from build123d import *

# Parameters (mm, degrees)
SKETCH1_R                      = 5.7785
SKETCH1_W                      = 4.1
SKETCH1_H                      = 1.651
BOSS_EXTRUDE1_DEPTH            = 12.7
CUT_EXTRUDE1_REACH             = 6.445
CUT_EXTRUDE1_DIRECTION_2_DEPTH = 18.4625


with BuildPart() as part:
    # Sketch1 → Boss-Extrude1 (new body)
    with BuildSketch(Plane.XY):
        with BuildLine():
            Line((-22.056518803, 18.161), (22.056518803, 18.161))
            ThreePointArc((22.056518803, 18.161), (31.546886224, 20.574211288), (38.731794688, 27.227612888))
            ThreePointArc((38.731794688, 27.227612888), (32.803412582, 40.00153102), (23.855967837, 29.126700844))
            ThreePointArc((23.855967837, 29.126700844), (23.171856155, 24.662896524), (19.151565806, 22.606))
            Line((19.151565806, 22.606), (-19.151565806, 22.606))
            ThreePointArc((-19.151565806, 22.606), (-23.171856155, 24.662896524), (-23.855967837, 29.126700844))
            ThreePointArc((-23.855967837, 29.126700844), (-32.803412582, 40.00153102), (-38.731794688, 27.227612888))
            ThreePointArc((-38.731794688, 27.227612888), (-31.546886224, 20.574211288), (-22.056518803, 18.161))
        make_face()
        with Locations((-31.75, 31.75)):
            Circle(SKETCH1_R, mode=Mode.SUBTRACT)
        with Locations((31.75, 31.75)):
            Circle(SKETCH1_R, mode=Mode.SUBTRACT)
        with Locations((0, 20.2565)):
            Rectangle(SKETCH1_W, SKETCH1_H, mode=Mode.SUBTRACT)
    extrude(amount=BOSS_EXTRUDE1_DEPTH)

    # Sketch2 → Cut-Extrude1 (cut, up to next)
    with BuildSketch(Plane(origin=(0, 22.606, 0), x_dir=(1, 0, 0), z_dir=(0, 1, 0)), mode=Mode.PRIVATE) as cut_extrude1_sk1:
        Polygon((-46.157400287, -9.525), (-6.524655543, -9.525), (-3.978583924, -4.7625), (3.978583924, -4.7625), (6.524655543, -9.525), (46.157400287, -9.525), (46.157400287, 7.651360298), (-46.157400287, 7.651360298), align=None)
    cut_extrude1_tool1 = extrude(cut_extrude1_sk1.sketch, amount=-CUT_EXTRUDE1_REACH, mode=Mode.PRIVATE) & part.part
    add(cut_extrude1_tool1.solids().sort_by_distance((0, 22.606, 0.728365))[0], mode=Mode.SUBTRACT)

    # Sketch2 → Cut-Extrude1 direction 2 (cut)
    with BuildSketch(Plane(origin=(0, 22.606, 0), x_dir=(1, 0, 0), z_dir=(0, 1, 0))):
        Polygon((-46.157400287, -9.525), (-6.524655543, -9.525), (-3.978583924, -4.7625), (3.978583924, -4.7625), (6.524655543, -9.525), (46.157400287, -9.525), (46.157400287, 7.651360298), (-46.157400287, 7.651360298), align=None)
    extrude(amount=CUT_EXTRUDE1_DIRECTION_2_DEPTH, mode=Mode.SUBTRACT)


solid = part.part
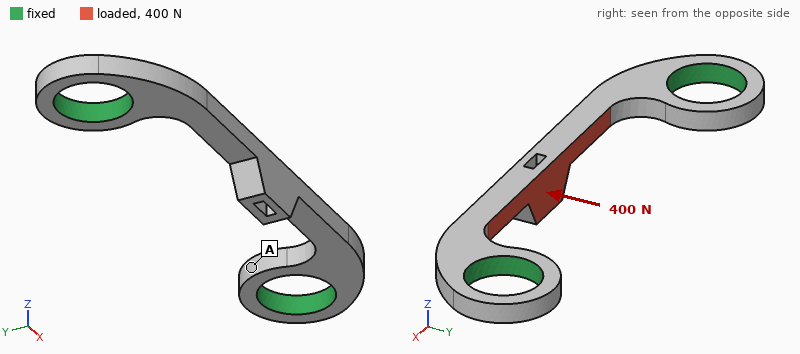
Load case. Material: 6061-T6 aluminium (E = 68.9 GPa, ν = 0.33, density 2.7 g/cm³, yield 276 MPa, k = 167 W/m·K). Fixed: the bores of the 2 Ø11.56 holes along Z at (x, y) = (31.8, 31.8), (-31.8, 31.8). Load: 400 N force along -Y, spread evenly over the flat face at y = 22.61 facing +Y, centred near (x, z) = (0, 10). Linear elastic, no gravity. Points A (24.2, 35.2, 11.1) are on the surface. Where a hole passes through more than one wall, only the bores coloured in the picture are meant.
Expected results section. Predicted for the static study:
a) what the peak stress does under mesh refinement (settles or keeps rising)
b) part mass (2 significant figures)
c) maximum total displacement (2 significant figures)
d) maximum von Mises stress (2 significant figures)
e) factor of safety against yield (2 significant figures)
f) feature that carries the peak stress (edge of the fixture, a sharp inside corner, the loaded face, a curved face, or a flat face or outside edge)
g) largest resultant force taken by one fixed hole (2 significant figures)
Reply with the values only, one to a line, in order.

settles
5.2 g
0.15 mm
170 MPa
1.7
a curved face
270 N
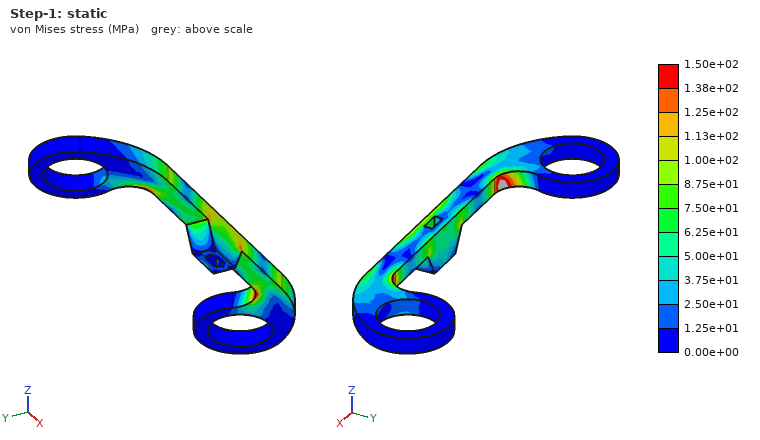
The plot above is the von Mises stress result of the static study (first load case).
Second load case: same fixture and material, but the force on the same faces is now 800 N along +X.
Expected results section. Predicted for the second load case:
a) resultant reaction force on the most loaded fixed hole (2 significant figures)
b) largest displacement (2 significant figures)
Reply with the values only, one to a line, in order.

400 N
30 µm
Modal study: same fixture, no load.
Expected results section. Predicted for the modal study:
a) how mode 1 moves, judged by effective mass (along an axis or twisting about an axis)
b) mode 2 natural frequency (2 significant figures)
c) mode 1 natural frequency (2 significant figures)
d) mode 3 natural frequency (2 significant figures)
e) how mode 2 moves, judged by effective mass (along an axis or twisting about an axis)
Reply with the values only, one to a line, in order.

along Z
7400 Hz
4800 Hz
12 kHz
along Y
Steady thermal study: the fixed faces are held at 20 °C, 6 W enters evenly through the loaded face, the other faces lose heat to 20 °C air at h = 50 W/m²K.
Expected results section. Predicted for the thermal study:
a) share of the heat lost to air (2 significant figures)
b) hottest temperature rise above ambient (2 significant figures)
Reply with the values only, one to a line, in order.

11 %
23 K
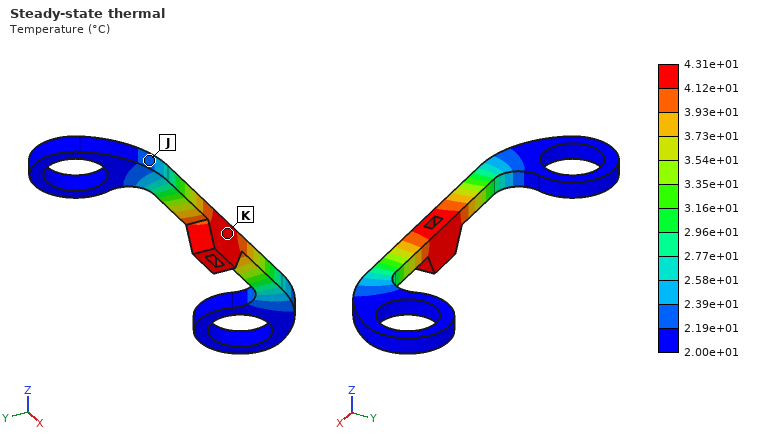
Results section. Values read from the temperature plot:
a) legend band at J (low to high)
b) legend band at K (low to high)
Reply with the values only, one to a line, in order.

2.19e+01 to 2.39e+01 °C
4.12e+01 to 4.31e+01 °C
